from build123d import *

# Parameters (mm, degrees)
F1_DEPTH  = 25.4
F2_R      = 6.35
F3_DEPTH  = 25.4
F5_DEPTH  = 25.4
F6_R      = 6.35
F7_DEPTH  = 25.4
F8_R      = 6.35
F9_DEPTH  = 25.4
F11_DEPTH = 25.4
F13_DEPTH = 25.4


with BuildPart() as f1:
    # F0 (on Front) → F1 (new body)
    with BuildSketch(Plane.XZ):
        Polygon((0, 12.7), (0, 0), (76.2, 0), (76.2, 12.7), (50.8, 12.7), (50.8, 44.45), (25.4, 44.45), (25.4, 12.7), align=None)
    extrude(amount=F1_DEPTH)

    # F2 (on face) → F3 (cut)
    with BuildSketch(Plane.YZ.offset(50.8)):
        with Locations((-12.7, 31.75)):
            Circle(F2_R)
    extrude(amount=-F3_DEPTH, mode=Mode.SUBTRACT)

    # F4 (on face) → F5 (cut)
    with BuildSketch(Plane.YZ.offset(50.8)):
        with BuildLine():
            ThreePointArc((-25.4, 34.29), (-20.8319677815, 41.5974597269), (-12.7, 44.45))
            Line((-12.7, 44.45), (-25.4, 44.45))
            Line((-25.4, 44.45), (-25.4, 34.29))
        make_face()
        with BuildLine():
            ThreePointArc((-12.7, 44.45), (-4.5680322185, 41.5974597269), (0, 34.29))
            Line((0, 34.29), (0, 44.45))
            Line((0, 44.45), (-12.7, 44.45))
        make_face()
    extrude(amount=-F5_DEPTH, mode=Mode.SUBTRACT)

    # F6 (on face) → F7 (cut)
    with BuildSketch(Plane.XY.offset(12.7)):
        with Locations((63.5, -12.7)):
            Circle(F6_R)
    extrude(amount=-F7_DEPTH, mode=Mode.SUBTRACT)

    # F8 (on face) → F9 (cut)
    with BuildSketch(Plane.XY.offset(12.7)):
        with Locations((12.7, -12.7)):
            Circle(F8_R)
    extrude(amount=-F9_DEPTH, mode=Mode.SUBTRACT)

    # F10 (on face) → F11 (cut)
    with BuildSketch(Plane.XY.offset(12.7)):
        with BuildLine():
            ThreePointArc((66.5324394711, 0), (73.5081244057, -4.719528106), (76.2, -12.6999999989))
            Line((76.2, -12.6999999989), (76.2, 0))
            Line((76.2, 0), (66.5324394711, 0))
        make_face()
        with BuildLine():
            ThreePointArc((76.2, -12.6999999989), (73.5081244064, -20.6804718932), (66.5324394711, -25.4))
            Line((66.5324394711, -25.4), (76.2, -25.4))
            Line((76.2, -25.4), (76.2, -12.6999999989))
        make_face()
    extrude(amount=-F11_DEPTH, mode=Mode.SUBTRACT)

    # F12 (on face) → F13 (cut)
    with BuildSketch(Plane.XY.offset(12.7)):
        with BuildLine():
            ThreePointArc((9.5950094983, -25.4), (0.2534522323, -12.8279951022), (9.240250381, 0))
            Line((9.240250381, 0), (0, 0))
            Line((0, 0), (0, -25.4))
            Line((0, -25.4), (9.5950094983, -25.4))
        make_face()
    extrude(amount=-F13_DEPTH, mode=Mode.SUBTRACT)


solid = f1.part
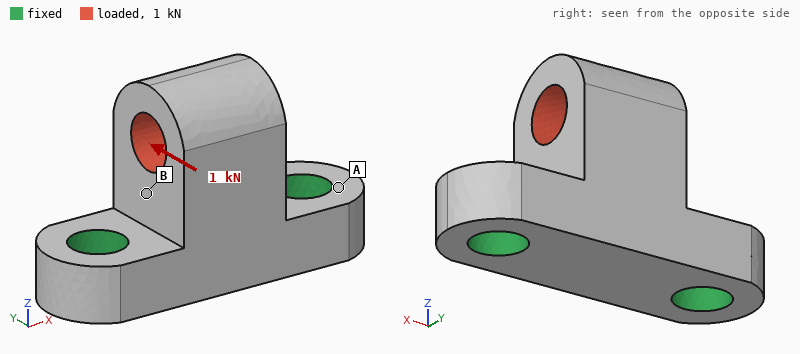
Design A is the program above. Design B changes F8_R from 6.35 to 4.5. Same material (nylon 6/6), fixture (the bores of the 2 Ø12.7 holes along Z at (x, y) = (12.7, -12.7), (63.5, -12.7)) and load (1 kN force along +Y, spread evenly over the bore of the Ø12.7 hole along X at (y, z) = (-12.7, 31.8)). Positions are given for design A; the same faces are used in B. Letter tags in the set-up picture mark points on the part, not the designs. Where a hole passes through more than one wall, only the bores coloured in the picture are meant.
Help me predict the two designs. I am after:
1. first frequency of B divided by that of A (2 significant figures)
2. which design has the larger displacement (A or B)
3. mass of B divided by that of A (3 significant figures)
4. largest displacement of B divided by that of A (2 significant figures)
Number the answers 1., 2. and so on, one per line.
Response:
1. 0.95
2. B
3. 1.02
4. 1.1
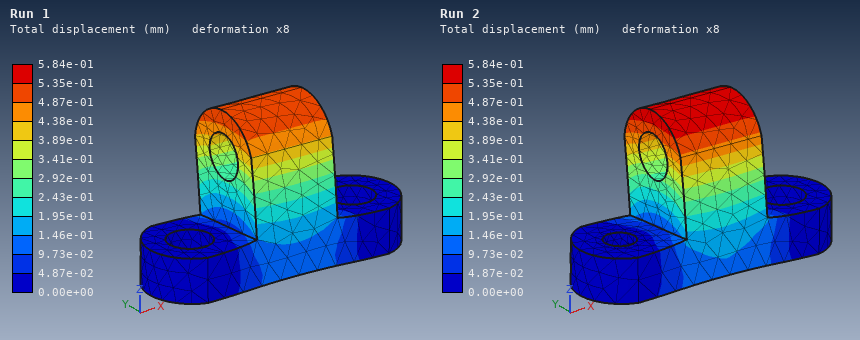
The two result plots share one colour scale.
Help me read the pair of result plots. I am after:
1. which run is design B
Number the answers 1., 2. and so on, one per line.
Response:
1. Run 2
